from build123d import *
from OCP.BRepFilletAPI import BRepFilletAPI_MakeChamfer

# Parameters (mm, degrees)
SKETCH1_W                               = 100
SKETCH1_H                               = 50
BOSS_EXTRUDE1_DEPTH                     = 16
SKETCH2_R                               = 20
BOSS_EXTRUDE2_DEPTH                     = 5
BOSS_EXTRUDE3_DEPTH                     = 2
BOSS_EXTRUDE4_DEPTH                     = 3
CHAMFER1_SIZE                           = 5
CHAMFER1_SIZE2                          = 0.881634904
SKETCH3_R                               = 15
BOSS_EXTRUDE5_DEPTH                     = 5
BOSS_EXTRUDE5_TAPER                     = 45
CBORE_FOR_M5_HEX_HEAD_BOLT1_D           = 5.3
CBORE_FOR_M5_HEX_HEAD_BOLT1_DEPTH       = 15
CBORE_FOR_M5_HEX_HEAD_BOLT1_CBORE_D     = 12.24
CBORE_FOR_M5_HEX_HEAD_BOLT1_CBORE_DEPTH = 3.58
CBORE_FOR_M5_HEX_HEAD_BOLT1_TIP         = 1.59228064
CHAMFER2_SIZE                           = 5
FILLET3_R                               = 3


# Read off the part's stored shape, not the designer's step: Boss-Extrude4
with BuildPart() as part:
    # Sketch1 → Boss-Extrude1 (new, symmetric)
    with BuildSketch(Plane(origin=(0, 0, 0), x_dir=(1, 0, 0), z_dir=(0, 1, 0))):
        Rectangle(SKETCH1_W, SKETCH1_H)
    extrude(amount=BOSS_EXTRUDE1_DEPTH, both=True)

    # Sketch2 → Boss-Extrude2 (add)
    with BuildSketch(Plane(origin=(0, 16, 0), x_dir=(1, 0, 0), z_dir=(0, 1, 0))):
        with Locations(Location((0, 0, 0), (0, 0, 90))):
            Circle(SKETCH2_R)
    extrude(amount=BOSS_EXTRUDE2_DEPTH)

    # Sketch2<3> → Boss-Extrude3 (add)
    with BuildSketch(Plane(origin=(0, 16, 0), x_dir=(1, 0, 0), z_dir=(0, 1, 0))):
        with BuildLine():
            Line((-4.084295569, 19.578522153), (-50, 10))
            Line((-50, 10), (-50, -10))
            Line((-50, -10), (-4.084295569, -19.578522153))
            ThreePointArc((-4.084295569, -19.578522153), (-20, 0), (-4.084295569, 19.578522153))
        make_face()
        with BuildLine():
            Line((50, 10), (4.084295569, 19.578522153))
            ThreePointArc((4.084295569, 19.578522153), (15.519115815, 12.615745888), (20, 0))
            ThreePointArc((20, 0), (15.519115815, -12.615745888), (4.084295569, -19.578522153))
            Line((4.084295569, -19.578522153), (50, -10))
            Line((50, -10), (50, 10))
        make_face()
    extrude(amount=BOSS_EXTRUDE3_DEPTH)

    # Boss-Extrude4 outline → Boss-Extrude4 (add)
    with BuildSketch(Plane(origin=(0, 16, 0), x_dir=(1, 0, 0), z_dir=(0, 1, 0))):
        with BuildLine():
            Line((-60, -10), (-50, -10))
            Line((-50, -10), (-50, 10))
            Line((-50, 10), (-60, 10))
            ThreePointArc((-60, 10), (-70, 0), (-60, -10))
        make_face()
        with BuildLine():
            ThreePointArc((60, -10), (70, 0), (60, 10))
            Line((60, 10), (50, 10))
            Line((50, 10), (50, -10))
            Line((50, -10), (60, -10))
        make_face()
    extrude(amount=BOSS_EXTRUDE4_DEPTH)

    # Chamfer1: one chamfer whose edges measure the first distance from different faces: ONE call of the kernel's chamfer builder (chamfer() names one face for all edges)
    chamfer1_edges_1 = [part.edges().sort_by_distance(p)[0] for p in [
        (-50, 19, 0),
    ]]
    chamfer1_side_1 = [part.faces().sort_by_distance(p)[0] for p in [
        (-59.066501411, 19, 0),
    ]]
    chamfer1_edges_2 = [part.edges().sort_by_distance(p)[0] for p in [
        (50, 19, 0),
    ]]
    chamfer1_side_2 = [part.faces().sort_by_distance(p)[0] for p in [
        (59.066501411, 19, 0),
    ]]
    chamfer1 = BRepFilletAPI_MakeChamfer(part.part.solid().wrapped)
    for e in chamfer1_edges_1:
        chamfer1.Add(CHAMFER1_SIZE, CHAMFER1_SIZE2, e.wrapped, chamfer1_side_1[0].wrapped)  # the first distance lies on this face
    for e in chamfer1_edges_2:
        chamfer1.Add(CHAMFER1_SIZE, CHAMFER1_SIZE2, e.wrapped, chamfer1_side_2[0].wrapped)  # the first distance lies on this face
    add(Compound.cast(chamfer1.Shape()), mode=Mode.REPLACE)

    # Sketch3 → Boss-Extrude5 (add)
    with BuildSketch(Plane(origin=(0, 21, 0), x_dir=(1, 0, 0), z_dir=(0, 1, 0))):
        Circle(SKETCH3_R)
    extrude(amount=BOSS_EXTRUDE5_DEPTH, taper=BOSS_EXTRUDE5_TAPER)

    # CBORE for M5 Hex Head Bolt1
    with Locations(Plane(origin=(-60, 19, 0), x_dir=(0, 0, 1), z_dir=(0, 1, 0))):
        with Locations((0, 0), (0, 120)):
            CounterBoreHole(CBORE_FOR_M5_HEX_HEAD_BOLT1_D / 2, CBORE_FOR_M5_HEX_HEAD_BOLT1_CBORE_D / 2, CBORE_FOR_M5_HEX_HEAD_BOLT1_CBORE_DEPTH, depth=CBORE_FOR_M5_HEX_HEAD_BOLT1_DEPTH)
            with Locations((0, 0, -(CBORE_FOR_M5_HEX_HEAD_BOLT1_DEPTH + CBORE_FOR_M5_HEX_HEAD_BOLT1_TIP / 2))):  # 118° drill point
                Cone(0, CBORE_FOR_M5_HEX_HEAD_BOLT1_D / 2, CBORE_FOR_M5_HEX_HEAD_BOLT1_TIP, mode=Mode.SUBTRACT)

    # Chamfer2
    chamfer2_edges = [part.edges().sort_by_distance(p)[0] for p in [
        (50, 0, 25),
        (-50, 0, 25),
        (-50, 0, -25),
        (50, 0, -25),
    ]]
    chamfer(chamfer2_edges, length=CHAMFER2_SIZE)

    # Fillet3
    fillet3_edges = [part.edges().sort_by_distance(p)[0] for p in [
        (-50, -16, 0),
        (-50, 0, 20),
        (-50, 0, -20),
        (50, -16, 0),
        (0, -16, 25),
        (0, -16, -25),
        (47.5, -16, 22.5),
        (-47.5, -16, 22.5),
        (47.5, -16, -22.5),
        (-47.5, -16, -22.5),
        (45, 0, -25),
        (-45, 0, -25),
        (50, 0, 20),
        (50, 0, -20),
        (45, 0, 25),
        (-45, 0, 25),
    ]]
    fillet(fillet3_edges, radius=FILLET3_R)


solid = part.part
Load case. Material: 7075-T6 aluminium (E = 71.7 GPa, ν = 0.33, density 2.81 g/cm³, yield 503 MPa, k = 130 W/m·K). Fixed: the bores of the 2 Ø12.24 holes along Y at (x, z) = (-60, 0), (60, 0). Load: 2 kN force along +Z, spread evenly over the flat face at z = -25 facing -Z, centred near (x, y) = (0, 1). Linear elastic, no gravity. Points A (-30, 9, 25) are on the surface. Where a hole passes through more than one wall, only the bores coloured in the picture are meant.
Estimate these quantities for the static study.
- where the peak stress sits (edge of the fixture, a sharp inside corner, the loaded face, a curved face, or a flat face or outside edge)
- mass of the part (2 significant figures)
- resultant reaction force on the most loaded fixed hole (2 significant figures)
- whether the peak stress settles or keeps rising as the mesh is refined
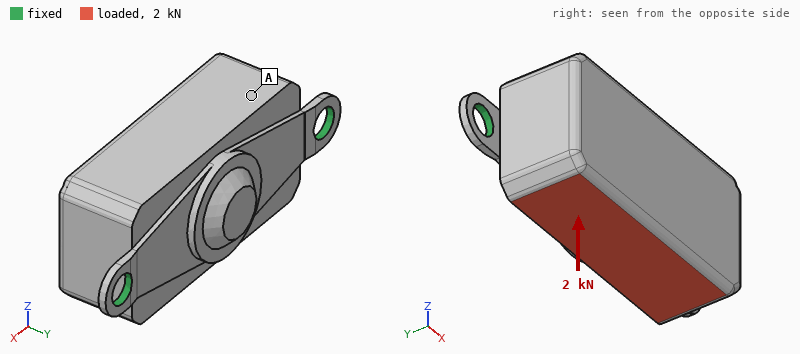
edge of the fixture
480 g
1.0 kN
keeps rising
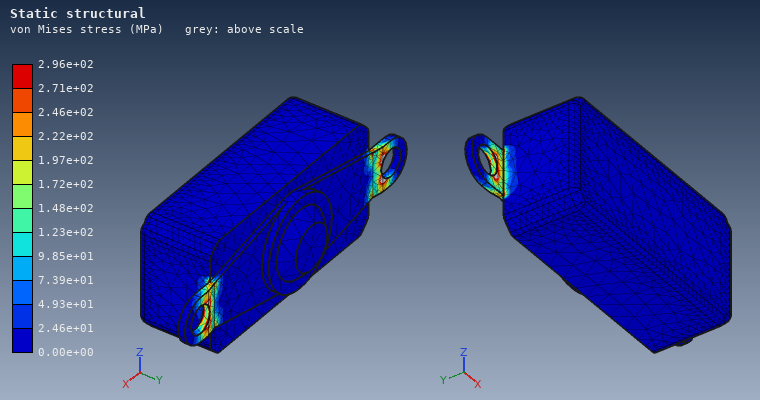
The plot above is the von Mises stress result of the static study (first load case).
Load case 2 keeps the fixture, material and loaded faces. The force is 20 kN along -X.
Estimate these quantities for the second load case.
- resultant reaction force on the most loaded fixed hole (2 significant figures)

11 kN
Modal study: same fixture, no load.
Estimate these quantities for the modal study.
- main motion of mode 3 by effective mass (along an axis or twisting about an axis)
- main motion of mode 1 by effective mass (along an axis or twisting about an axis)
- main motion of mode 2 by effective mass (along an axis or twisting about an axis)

along X
along Z
along Y
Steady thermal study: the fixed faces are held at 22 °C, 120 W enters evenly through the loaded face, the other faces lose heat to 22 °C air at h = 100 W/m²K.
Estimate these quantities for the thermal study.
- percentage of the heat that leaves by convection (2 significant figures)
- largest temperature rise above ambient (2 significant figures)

56 %
47 K
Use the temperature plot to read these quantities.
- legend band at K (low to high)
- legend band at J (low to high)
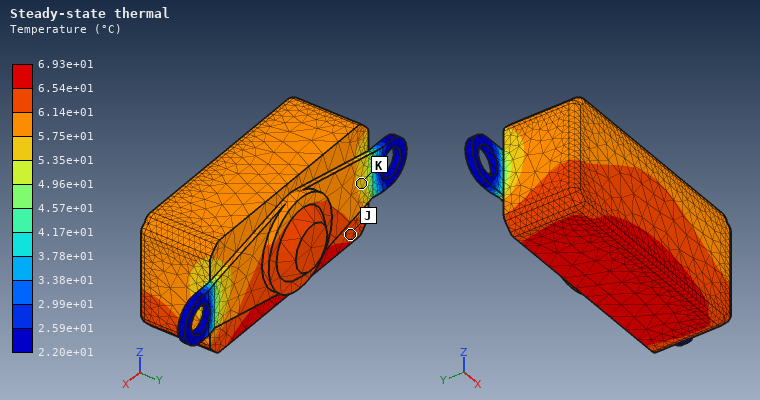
5.35e+01 to 5.75e+01 °C
6.14e+01 to 6.54e+01 °C
